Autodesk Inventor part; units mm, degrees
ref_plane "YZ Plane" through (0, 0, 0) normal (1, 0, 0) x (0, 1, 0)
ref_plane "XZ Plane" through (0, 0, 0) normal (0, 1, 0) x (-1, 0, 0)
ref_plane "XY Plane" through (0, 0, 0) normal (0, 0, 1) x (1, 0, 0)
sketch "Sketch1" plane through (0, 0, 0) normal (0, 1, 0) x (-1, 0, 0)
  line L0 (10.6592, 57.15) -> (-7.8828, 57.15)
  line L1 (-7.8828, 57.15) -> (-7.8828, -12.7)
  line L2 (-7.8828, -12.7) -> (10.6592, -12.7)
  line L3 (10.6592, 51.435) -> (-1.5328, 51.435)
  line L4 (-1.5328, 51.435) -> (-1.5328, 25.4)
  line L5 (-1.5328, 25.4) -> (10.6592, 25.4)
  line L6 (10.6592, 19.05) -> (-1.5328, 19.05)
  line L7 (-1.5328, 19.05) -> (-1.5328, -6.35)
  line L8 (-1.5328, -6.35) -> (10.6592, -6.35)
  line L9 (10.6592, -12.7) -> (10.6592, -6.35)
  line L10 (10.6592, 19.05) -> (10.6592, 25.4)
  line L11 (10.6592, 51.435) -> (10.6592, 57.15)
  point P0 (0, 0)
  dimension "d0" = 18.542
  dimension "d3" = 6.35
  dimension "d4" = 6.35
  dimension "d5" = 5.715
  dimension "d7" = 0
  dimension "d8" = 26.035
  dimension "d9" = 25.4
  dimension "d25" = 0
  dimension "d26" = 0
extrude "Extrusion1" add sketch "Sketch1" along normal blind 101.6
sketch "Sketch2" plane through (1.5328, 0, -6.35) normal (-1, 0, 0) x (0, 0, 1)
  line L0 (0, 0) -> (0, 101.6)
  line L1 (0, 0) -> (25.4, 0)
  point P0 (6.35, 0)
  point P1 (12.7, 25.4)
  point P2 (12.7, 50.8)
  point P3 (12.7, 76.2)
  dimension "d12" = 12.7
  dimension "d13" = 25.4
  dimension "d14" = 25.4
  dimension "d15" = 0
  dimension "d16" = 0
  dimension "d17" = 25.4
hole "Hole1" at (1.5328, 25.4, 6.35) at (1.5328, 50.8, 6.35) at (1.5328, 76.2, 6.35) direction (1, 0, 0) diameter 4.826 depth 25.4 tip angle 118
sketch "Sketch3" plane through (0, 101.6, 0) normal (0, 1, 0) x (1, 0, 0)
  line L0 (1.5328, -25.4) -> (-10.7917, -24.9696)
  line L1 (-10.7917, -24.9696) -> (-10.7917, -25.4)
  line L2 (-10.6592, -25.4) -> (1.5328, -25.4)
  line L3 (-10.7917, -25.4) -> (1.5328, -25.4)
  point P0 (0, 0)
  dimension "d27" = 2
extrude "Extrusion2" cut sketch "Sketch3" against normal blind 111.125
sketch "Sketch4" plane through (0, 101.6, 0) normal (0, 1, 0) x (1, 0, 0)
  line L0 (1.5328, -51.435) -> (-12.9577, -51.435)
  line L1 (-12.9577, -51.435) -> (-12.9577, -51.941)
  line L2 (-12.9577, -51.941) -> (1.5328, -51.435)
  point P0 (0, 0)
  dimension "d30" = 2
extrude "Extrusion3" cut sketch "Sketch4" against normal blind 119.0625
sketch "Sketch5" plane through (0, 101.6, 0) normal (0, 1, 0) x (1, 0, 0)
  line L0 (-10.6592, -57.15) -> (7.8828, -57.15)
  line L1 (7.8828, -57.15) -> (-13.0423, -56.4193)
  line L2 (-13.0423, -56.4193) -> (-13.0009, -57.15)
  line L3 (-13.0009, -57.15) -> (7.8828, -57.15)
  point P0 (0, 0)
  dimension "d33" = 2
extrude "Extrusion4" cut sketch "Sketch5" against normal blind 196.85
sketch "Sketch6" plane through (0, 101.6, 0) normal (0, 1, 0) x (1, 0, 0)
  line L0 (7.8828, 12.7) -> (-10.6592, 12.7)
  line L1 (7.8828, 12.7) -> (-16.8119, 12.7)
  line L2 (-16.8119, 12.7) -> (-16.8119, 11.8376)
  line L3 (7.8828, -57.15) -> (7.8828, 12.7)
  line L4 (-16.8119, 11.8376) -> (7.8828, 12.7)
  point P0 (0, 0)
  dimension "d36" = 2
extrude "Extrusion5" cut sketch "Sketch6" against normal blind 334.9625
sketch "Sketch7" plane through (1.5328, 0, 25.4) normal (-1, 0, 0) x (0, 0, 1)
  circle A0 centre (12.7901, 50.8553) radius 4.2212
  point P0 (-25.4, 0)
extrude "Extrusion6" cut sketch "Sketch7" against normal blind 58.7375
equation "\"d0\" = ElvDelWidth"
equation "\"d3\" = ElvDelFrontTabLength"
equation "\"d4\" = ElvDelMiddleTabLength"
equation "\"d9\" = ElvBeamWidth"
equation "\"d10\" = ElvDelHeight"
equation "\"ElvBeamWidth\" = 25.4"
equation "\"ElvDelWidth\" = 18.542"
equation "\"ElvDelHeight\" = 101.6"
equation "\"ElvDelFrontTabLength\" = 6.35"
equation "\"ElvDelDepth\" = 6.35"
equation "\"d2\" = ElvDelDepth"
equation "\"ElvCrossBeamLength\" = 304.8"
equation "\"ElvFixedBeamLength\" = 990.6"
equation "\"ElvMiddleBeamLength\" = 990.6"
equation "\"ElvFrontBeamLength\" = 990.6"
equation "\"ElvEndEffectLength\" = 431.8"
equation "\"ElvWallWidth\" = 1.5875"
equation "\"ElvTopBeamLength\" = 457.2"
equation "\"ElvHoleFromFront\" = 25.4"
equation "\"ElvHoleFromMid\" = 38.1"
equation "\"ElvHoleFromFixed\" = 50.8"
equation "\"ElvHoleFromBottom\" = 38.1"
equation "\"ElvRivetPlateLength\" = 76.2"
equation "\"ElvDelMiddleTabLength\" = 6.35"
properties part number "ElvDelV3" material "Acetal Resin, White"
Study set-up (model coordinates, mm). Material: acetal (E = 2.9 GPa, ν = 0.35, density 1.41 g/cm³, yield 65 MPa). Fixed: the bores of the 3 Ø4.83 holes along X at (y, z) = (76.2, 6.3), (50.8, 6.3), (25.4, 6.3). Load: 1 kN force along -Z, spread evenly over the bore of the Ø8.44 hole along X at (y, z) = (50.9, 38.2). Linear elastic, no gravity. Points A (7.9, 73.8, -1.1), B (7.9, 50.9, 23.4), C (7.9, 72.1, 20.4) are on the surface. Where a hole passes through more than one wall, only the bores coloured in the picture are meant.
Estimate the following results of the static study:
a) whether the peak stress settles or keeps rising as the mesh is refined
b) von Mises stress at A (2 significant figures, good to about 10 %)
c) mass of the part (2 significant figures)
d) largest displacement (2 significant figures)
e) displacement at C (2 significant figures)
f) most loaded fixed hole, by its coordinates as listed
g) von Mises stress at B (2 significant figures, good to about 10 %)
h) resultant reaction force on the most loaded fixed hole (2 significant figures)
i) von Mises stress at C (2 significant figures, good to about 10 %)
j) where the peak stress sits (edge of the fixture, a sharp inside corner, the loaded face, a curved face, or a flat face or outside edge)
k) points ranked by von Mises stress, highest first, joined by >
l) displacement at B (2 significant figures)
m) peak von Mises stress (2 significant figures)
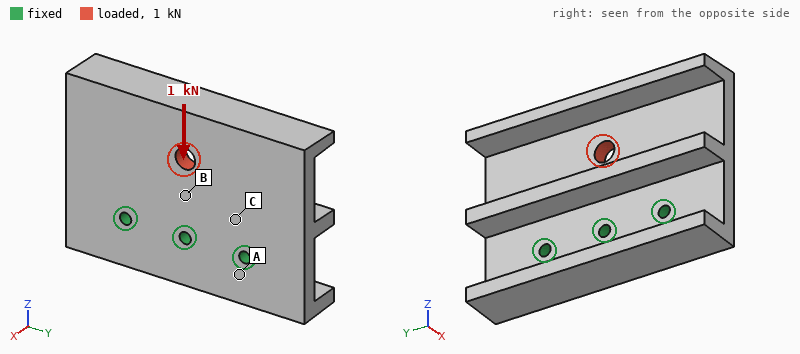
settles
1.1 MPa
92 g
60 µm
13 µm
(50.8, 6.3)
4.4 MPa
420 N
2.3 MPa
the loaded face
B > C > A
24 µm
12 MPa
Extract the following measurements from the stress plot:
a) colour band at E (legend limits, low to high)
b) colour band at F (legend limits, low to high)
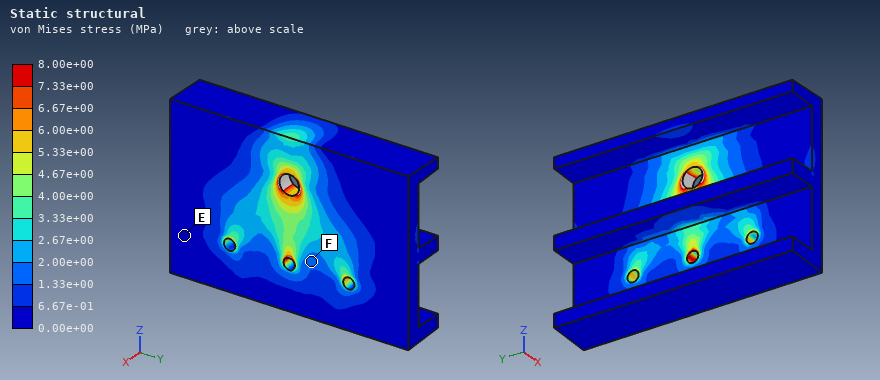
0.00e+00 to 6.67e-01 MPa
1.33e+00 to 2.00e+00 MPa
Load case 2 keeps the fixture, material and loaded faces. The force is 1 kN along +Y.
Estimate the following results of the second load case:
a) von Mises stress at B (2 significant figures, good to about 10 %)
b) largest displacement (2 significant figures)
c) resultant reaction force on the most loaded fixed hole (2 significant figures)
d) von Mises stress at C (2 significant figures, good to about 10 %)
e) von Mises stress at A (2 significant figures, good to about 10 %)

4.7 MPa
0.14 mm
680 N
4.2 MPa
2.3 MPa
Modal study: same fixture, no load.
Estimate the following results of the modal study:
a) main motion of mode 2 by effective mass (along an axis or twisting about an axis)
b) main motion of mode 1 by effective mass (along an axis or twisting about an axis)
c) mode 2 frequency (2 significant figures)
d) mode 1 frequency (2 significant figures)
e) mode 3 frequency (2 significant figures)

twisting about Z
along X
640 Hz
420 Hz
1700 Hz
